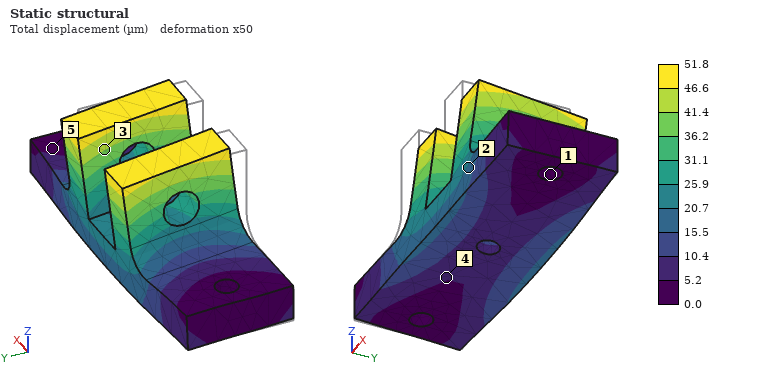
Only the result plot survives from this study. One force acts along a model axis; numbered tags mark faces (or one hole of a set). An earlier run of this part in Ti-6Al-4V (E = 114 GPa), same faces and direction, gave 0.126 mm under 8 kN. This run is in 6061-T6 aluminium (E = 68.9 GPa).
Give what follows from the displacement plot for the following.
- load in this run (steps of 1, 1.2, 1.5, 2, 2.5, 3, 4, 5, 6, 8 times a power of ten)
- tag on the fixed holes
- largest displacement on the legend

2 kN
1
51.8 µm
